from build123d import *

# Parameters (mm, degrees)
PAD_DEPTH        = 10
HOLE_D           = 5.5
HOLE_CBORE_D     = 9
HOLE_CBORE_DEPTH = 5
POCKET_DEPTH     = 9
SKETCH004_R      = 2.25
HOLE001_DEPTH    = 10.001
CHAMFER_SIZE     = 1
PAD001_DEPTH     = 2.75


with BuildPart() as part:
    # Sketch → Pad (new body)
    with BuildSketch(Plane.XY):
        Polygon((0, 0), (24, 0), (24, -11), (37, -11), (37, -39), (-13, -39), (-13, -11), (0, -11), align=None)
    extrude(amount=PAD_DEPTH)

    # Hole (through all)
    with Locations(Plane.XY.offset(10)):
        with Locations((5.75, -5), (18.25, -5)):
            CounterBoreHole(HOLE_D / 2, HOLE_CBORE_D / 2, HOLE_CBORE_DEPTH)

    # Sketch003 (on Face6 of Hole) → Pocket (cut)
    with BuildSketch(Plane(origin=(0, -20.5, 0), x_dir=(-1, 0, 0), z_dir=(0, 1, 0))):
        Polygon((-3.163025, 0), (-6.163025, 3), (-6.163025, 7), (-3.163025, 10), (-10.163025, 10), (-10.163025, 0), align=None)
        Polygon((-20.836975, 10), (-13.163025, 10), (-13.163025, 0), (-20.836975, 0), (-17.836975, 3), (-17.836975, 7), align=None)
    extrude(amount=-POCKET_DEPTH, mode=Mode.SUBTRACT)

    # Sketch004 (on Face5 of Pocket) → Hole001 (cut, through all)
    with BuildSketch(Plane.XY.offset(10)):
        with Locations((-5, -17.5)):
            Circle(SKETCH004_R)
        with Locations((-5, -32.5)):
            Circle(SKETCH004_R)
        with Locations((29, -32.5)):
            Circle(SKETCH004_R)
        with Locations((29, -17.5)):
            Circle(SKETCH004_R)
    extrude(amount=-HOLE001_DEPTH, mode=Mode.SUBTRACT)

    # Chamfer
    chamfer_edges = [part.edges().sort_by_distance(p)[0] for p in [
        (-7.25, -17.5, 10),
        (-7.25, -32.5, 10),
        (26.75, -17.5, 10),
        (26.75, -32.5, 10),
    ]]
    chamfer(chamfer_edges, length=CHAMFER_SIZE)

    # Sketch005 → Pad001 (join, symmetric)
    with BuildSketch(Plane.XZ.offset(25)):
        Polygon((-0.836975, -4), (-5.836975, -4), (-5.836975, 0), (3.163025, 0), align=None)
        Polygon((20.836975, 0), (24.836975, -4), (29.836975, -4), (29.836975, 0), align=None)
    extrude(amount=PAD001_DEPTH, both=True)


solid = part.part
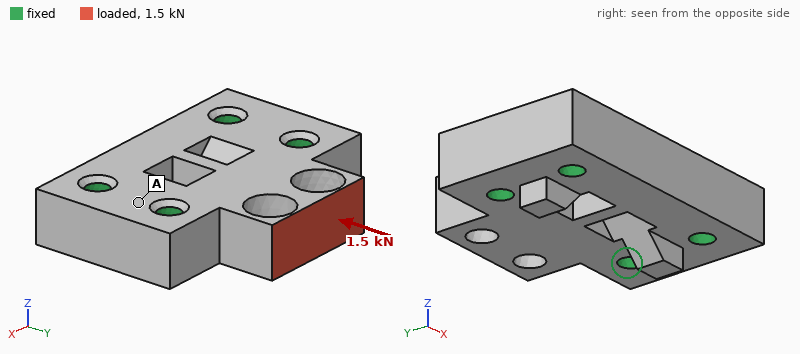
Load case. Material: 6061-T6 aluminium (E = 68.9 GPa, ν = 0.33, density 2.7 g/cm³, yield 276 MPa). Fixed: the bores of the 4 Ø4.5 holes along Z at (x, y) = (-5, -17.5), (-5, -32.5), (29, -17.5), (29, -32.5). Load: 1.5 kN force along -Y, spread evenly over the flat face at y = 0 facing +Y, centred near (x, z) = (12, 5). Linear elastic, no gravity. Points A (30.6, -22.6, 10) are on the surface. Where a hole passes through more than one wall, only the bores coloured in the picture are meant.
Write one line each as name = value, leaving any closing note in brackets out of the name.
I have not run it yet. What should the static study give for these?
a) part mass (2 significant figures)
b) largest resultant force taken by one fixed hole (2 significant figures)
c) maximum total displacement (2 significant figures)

part mass = 39 g
largest resultant force taken by one fixed hole = 510 N
maximum total displacement = 15 µm
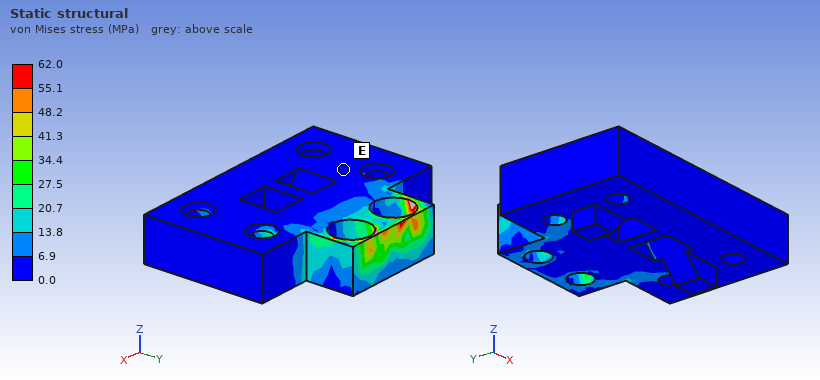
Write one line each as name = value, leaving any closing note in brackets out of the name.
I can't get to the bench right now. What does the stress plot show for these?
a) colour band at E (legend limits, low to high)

colour band at E = 0.0 to 6.9 MPa
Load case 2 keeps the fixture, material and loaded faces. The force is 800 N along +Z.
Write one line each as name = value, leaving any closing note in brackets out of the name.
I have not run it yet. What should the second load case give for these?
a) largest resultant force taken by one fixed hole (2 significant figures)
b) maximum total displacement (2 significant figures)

largest resultant force taken by one fixed hole = 580 N
maximum total displacement = 31 µm
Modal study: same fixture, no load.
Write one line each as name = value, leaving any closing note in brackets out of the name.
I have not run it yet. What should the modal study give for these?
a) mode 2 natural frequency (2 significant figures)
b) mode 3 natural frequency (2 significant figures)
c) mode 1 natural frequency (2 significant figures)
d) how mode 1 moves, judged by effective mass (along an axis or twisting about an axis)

mode 2 natural frequency = 31 kHz
mode 3 natural frequency = 32 kHz
mode 1 natural frequency = 18 kHz
how mode 1 moves, judged by effective mass = along Z
